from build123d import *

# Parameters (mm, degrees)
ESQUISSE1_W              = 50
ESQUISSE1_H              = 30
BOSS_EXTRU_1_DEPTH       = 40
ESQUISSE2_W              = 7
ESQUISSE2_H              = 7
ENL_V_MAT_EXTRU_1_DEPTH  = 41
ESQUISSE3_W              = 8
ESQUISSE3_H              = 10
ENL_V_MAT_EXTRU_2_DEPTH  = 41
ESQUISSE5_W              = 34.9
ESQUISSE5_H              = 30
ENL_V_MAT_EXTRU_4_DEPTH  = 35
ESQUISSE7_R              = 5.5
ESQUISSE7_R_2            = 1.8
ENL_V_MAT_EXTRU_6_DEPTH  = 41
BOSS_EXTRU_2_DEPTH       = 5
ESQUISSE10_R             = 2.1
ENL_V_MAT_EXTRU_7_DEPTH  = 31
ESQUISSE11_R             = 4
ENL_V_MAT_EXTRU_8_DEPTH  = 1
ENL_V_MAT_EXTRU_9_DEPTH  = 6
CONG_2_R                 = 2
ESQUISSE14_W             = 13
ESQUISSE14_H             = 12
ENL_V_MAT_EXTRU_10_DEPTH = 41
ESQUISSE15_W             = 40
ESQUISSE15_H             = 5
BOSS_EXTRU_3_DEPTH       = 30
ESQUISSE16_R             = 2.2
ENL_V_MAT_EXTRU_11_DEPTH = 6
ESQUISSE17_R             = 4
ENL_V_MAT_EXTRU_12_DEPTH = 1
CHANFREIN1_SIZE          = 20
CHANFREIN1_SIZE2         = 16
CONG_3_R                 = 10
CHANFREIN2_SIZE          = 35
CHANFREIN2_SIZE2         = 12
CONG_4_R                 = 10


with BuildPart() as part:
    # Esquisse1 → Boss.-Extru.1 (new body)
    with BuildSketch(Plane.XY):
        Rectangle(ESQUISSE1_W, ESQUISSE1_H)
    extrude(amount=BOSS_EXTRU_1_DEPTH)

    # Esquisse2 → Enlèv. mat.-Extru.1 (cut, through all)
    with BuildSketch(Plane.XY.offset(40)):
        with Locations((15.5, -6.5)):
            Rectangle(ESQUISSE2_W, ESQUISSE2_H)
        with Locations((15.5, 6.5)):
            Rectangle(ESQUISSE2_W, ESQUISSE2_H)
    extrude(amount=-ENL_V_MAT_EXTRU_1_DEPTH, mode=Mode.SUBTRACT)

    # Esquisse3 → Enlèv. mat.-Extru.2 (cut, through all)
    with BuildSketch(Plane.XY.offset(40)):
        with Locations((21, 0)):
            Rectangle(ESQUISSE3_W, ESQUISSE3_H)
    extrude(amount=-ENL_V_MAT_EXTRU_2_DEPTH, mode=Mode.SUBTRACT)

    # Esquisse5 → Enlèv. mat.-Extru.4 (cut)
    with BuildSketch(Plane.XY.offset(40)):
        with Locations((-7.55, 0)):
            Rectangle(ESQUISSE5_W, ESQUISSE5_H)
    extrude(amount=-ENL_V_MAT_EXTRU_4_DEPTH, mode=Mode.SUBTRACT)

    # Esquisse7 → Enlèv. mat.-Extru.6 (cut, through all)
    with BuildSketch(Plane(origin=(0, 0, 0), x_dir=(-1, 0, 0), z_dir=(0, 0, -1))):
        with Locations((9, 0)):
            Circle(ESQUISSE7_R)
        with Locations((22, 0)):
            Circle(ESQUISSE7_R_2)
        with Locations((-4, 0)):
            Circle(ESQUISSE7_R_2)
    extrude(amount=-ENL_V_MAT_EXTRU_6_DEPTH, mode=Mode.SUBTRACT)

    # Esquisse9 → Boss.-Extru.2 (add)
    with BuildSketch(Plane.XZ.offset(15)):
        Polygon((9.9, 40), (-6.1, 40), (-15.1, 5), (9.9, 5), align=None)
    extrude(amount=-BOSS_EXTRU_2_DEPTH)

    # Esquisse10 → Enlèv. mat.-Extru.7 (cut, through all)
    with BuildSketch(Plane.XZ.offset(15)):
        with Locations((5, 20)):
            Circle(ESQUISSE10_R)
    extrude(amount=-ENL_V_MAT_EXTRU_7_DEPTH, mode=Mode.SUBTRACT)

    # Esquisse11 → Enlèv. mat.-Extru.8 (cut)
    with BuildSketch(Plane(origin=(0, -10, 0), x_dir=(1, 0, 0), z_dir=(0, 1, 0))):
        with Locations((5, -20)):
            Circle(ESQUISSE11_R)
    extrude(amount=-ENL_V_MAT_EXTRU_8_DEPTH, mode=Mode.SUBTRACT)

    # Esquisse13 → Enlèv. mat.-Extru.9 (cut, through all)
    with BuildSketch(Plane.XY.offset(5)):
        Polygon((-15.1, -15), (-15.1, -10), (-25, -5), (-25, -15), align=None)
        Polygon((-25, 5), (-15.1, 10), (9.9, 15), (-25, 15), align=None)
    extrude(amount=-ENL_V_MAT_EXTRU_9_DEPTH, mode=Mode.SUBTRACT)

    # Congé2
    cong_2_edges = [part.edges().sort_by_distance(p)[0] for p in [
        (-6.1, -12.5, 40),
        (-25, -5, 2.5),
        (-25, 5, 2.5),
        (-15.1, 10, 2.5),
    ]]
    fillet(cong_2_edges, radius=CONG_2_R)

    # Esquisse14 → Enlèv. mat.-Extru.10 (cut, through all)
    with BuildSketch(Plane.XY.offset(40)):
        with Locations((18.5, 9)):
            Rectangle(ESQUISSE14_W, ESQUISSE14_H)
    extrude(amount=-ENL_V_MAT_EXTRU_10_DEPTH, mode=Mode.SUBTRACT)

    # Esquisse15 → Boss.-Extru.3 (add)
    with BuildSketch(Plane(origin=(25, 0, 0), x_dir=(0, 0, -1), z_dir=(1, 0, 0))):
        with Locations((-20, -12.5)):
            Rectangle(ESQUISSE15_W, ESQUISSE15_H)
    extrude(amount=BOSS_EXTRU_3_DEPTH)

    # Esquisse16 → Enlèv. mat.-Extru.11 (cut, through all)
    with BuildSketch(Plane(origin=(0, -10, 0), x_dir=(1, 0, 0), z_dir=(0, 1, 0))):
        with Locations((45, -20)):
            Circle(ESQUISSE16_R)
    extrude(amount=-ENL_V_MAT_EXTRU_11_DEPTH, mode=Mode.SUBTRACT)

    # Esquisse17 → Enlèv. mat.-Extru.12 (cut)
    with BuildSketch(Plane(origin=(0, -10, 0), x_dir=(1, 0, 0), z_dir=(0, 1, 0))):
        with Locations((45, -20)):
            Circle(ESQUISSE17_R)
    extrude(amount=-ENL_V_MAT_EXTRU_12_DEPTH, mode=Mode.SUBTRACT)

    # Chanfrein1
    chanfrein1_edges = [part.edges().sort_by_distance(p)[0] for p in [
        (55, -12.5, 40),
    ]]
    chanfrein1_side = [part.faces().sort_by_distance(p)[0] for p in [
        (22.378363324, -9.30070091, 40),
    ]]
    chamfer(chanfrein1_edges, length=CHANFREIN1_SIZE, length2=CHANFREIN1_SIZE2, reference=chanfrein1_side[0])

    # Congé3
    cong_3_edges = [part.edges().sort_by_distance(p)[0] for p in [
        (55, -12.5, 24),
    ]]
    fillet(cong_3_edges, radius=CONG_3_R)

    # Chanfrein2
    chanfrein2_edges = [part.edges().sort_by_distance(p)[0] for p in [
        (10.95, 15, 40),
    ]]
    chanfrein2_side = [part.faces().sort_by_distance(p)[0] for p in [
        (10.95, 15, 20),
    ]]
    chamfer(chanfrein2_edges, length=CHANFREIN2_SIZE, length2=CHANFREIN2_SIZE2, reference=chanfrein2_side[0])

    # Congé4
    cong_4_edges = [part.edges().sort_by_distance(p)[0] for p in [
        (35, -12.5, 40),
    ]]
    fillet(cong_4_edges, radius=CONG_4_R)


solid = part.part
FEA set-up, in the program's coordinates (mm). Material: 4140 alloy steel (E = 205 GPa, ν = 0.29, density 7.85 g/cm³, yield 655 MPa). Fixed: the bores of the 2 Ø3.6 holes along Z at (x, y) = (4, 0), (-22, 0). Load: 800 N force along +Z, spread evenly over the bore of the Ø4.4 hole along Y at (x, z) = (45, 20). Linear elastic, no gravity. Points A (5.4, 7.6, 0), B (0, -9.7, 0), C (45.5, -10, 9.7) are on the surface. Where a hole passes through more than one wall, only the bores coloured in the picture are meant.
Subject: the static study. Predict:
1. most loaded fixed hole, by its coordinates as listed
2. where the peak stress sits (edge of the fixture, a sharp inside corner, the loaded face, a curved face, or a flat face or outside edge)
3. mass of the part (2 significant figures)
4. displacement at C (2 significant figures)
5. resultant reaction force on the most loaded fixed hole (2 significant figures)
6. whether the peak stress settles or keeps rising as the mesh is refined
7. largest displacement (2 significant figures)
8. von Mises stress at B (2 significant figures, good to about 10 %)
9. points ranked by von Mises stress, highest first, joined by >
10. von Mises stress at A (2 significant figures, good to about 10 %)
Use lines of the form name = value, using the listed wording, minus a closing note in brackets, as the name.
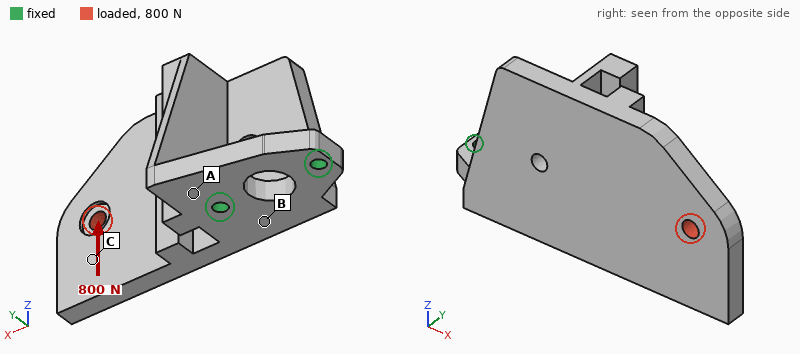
most loaded fixed hole, by its coordinates as listed = (4, 0)
where the peak stress sits = edge of the fixture
mass of the part = 150 g
displacement at C = 0.11 mm
resultant reaction force on the most loaded fixed hole = 1.8 kN
whether the peak stress settles or keeps rising as the mesh is refined = keeps rising
largest displacement = 0.15 mm
von Mises stress at B = 85 MPa
points ranked by von Mises stress, highest first, joined by > = B > A > C
von Mises stress at A = 53 MPa
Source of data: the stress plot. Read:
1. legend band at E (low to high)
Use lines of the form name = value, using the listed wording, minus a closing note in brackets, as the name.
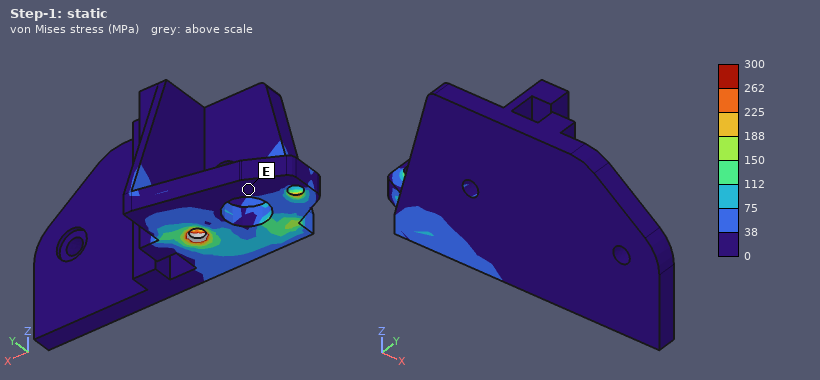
legend band at E = 0 to 38 MPa
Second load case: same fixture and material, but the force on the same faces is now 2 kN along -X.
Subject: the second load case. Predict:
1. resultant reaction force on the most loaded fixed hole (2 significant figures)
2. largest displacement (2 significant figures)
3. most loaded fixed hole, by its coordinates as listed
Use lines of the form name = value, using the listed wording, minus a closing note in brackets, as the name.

resultant reaction force on the most loaded fixed hole = 1.8 kN
largest displacement = 0.11 mm
most loaded fixed hole, by its coordinates as listed = (4, 0)
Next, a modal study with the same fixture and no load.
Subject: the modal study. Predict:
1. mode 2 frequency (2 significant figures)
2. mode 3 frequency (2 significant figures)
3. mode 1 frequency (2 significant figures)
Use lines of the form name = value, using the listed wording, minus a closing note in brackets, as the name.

mode 2 frequency = 2000 Hz
mode 3 frequency = 2900 Hz
mode 1 frequency = 1400 Hz
